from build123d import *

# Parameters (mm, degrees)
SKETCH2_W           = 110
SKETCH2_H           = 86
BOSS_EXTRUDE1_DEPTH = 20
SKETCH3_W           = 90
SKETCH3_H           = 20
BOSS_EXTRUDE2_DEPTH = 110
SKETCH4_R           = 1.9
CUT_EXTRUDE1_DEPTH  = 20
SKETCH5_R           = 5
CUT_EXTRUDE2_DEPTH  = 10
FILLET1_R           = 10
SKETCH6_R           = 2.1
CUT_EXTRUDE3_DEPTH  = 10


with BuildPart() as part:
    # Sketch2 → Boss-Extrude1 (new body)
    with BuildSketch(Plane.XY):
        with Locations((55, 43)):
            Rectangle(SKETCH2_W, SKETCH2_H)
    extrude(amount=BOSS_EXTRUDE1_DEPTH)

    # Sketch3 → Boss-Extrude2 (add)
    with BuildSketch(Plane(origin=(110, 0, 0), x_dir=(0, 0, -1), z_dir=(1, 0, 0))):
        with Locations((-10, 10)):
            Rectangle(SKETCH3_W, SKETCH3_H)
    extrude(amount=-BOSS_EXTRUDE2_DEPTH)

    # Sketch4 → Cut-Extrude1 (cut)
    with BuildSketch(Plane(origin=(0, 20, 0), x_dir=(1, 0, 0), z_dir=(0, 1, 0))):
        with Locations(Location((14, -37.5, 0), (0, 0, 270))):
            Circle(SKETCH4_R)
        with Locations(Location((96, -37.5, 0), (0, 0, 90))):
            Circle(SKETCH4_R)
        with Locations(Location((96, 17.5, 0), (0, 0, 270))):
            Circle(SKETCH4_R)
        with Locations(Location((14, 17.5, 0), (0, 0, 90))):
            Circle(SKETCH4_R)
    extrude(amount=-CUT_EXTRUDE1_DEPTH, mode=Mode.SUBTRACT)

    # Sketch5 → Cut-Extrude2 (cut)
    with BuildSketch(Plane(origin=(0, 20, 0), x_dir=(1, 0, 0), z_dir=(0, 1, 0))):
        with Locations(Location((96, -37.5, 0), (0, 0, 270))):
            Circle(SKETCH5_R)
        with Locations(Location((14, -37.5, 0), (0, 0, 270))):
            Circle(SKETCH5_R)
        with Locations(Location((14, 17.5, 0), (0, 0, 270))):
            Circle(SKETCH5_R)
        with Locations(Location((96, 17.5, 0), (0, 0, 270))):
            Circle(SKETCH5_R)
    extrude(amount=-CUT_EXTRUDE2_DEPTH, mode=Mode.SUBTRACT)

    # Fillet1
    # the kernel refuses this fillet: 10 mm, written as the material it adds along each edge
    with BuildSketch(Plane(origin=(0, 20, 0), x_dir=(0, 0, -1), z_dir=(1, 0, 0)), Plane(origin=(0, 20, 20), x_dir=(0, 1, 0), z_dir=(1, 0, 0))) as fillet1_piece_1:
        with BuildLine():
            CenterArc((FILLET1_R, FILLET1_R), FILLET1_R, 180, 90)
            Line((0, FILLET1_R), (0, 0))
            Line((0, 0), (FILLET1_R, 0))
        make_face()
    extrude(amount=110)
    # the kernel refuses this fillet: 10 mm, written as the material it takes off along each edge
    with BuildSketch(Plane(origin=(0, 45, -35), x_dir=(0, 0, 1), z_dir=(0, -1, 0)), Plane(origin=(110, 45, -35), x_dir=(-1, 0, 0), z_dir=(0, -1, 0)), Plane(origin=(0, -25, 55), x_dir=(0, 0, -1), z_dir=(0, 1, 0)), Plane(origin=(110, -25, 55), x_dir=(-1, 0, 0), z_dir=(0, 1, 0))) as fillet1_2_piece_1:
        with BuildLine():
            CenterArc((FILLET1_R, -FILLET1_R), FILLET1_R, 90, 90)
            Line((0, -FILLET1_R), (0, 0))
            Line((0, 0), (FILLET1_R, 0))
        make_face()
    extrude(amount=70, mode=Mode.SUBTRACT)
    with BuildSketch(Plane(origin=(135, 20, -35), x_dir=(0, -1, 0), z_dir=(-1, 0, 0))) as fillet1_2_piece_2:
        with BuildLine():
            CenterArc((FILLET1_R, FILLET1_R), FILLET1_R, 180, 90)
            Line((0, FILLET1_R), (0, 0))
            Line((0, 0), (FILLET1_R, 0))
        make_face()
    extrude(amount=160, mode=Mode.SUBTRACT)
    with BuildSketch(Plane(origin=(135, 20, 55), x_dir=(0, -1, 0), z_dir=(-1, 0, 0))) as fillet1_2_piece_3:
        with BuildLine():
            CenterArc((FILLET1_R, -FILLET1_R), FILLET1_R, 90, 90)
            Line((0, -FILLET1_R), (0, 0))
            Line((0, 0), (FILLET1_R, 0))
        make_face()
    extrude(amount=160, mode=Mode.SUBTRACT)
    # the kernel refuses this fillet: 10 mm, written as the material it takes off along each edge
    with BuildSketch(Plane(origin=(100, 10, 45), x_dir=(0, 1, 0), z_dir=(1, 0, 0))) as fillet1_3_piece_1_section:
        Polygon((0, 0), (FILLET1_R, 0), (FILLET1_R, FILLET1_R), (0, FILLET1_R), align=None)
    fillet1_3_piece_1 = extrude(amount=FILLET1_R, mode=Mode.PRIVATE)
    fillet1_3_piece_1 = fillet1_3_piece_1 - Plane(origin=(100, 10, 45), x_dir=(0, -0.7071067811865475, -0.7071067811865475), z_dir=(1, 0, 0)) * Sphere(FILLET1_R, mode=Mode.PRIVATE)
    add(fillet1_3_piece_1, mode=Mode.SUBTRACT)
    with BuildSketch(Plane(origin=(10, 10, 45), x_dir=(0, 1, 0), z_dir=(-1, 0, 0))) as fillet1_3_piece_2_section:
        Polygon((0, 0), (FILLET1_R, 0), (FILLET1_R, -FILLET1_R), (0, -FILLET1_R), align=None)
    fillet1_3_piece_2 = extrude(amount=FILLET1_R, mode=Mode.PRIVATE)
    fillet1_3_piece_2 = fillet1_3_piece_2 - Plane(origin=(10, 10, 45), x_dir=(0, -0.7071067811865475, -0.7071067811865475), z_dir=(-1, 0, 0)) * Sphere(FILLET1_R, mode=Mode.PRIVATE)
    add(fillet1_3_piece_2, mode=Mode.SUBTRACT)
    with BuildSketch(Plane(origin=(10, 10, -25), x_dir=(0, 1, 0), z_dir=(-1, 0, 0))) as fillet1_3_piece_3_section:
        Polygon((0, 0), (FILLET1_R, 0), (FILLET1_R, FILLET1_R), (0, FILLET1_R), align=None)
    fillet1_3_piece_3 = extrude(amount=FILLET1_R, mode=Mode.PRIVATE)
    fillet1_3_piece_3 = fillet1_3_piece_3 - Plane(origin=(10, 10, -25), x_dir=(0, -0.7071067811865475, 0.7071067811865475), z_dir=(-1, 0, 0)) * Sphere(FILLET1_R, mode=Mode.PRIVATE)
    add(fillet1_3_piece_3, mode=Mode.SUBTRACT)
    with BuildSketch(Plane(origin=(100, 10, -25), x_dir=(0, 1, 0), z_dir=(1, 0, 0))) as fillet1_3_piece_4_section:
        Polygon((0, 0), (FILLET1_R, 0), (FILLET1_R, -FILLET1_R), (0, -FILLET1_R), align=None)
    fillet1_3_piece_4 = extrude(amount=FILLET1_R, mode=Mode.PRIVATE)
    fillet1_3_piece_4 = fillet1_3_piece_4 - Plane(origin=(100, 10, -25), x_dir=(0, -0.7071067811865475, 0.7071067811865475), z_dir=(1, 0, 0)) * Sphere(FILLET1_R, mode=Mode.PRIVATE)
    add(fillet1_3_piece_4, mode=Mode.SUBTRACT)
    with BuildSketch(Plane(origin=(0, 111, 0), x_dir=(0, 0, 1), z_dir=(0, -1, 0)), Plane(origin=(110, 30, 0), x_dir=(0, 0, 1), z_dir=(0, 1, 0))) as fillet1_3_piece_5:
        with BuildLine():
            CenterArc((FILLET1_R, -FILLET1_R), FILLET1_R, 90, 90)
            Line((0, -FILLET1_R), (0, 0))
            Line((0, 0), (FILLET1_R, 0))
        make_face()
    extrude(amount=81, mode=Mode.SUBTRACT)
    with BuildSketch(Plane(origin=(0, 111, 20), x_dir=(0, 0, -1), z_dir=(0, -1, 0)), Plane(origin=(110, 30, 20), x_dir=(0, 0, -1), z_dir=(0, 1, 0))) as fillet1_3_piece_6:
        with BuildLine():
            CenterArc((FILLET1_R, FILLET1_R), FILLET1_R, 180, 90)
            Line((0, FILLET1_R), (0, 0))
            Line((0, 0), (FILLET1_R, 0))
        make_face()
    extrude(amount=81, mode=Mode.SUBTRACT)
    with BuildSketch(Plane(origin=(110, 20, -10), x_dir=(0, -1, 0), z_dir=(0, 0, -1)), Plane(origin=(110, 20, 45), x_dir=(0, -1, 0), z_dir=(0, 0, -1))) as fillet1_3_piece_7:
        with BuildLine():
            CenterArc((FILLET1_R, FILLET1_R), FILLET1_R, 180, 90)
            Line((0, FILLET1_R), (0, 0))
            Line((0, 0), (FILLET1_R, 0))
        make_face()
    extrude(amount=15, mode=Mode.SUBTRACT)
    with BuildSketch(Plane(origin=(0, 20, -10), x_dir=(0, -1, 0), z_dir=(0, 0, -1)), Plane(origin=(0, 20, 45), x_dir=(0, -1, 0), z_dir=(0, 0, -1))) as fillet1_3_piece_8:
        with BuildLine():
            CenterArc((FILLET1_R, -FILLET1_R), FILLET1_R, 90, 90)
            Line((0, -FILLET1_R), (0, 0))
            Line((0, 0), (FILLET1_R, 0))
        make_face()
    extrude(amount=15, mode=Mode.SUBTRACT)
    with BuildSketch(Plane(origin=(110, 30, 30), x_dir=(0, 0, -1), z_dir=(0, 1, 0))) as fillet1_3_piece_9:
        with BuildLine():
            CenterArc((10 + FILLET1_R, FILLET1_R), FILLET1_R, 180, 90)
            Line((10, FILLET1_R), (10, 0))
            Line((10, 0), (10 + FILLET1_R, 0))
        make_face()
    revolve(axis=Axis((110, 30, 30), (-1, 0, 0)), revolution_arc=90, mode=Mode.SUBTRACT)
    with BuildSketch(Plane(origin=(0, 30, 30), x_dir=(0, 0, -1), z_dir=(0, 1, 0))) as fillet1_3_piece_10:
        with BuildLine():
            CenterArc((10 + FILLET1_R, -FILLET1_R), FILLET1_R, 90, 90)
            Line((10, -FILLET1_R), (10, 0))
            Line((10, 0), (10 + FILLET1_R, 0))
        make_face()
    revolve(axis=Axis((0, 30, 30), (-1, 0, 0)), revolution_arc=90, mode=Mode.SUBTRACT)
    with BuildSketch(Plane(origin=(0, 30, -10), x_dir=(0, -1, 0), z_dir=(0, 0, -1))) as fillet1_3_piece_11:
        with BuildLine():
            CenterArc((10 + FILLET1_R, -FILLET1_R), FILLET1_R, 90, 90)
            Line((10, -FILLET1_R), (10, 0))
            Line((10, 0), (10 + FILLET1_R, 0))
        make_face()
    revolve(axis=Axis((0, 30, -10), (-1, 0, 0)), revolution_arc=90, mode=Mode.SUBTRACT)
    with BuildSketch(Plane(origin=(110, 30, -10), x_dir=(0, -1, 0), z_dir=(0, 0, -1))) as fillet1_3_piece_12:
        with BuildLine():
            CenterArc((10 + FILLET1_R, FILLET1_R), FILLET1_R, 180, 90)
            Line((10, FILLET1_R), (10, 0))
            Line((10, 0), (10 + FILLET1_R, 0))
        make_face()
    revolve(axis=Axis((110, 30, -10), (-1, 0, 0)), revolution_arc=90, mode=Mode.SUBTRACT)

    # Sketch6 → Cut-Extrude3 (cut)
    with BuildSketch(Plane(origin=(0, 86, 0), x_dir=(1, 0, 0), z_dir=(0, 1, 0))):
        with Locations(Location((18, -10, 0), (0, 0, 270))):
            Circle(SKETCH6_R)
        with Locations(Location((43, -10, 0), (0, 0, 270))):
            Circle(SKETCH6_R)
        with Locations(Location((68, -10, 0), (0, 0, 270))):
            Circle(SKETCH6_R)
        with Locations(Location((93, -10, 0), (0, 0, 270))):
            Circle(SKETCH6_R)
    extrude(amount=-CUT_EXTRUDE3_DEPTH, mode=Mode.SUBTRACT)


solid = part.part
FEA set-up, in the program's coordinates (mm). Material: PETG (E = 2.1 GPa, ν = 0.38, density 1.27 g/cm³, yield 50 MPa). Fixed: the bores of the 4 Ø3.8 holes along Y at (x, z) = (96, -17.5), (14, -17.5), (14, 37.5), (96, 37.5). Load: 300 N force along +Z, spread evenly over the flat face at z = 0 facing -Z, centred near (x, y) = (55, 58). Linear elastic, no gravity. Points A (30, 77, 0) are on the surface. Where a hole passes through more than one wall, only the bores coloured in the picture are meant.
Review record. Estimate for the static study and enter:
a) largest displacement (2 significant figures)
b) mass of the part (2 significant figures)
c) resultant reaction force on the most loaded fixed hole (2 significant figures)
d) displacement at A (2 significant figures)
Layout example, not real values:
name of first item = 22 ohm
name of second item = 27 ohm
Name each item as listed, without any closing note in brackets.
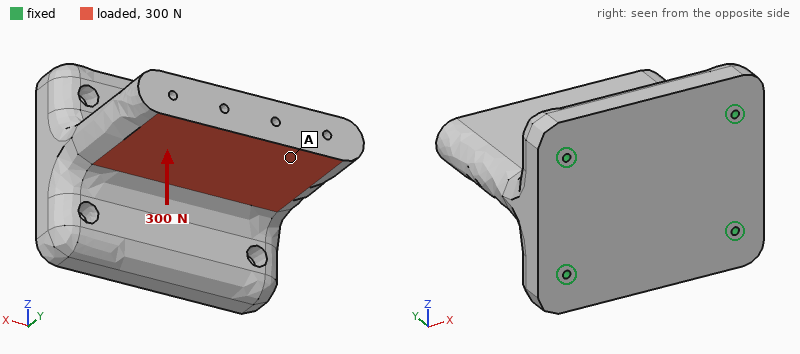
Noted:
largest displacement = 0.13 mm
mass of the part = 420 g
resultant reaction force on the most loaded fixed hole = 170 N
displacement at A = 0.11 mm
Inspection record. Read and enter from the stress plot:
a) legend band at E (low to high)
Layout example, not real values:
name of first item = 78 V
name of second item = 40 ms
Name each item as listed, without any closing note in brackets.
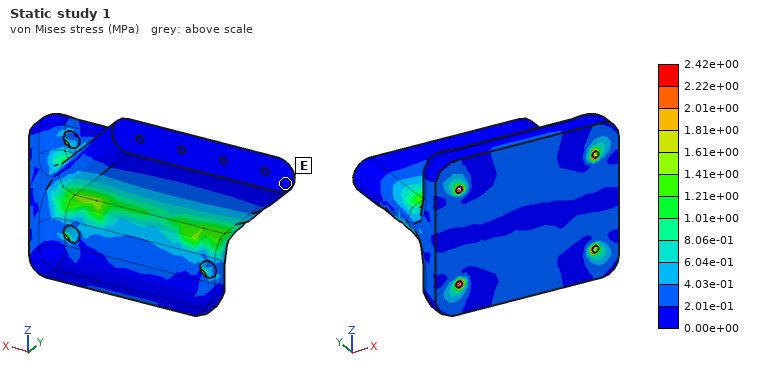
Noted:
legend band at E = 0.00e+00 to 2.01e-01 MPa
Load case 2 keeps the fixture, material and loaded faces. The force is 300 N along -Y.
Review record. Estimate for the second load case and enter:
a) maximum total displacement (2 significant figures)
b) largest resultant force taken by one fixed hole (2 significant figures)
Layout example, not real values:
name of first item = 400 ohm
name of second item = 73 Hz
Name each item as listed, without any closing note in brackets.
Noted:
maximum total displacement = 45 µm
largest resultant force taken by one fixed hole = 110 N
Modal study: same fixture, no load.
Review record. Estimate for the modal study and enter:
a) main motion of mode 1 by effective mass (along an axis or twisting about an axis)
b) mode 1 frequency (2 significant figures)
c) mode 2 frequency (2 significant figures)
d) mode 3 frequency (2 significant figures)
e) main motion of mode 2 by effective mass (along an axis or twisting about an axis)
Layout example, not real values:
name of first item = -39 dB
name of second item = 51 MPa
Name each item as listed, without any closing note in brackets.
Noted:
main motion of mode 1 by effective mass = along Z
mode 1 frequency = 770 Hz
mode 2 frequency = 1300 Hz
mode 3 frequency = 1300 Hz
main motion of mode 2 by effective mass = along X
